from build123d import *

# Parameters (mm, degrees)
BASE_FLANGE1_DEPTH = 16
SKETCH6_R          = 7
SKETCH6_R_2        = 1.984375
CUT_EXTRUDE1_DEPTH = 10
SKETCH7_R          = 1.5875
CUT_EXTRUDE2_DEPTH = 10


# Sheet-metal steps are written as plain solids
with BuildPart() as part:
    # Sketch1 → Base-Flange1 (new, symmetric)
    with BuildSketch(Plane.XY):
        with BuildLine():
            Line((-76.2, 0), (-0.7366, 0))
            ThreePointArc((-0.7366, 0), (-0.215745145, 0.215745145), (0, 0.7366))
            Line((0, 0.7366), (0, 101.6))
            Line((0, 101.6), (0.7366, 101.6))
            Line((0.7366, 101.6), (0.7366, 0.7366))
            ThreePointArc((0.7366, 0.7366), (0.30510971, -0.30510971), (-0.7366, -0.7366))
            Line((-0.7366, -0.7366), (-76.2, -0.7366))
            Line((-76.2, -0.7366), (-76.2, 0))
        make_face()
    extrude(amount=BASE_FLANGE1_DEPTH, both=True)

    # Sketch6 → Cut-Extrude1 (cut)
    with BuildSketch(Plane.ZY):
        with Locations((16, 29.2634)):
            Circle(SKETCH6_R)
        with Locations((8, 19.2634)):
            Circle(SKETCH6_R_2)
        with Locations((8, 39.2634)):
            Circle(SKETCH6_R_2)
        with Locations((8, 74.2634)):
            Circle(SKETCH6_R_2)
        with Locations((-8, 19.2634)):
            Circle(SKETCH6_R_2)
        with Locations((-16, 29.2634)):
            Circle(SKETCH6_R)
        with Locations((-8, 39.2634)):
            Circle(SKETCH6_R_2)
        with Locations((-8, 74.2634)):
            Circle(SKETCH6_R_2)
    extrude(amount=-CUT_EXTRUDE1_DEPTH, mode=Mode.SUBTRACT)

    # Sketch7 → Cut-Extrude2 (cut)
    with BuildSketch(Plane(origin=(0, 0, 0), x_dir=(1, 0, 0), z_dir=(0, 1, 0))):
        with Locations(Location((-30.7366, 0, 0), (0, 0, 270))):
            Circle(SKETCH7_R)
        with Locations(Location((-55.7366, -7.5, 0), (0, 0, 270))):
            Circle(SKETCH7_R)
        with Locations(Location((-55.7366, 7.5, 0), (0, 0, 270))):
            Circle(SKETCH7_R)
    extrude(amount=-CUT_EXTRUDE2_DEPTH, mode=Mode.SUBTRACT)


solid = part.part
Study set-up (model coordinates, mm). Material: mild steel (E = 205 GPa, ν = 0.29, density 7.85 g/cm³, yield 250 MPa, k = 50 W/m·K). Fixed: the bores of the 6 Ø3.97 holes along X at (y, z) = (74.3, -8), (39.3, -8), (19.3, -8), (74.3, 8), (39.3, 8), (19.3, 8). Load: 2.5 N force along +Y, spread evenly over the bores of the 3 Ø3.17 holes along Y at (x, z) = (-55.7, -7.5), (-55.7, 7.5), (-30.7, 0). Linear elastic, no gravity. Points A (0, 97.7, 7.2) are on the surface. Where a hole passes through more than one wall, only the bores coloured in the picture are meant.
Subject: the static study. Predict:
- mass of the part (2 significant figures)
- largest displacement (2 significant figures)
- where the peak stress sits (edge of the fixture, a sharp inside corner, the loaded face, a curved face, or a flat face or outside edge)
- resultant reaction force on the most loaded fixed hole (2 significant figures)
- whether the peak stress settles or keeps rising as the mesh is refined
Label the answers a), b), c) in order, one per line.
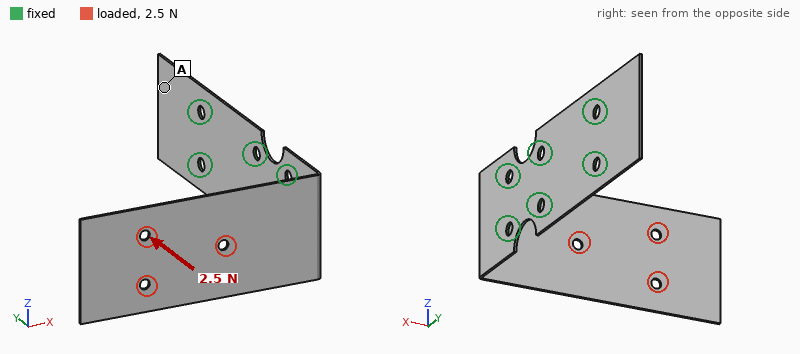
a) 31 g
b) 1.5 mm
c) edge of the fixture
d) 1.3 N
e) keeps rising
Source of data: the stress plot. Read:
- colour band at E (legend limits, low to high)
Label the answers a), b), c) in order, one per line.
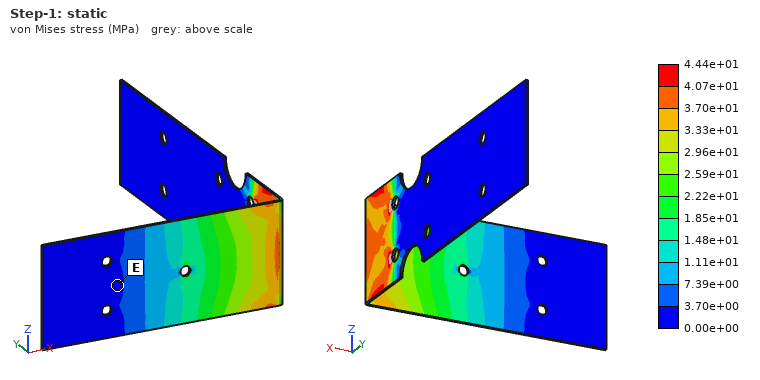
a) 0.00e+00 to 3.70e+00 MPa
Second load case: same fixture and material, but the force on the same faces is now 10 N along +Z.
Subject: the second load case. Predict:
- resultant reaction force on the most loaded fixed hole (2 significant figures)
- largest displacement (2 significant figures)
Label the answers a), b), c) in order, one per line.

a) 25 N
b) 1.0 mm
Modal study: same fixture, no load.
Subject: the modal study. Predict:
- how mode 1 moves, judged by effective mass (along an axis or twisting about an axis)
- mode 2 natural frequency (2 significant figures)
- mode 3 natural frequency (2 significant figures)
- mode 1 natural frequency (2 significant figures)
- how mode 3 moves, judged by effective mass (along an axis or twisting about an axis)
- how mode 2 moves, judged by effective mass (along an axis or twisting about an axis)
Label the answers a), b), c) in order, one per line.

a) along Y
b) 180 Hz
c) 440 Hz
d) 76 Hz
e) along X
f) along Z
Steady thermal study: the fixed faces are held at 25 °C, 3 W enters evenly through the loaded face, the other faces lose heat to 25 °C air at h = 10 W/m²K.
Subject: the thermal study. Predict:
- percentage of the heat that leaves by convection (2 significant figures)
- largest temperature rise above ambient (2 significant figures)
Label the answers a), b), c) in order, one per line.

a) 73 %
b) 63 K
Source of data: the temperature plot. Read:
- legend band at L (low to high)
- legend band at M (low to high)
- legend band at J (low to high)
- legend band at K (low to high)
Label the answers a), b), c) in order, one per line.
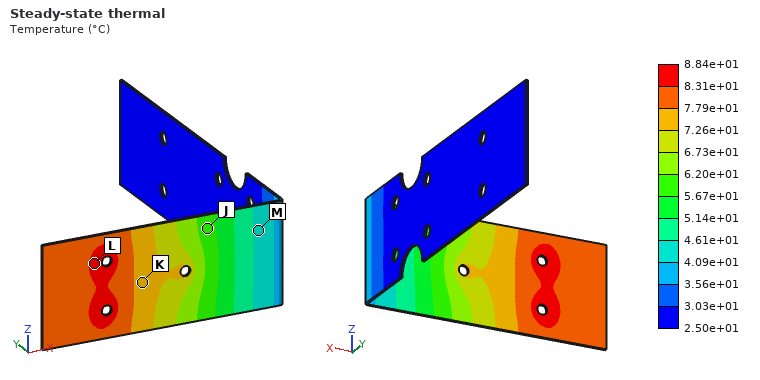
a) 8.31e+01 to 8.84e+01 °C
b) 4.09e+01 to 4.61e+01 °C
c) 5.67e+01 to 6.20e+01 °C
d) 7.26e+01 to 7.79e+01 °C
